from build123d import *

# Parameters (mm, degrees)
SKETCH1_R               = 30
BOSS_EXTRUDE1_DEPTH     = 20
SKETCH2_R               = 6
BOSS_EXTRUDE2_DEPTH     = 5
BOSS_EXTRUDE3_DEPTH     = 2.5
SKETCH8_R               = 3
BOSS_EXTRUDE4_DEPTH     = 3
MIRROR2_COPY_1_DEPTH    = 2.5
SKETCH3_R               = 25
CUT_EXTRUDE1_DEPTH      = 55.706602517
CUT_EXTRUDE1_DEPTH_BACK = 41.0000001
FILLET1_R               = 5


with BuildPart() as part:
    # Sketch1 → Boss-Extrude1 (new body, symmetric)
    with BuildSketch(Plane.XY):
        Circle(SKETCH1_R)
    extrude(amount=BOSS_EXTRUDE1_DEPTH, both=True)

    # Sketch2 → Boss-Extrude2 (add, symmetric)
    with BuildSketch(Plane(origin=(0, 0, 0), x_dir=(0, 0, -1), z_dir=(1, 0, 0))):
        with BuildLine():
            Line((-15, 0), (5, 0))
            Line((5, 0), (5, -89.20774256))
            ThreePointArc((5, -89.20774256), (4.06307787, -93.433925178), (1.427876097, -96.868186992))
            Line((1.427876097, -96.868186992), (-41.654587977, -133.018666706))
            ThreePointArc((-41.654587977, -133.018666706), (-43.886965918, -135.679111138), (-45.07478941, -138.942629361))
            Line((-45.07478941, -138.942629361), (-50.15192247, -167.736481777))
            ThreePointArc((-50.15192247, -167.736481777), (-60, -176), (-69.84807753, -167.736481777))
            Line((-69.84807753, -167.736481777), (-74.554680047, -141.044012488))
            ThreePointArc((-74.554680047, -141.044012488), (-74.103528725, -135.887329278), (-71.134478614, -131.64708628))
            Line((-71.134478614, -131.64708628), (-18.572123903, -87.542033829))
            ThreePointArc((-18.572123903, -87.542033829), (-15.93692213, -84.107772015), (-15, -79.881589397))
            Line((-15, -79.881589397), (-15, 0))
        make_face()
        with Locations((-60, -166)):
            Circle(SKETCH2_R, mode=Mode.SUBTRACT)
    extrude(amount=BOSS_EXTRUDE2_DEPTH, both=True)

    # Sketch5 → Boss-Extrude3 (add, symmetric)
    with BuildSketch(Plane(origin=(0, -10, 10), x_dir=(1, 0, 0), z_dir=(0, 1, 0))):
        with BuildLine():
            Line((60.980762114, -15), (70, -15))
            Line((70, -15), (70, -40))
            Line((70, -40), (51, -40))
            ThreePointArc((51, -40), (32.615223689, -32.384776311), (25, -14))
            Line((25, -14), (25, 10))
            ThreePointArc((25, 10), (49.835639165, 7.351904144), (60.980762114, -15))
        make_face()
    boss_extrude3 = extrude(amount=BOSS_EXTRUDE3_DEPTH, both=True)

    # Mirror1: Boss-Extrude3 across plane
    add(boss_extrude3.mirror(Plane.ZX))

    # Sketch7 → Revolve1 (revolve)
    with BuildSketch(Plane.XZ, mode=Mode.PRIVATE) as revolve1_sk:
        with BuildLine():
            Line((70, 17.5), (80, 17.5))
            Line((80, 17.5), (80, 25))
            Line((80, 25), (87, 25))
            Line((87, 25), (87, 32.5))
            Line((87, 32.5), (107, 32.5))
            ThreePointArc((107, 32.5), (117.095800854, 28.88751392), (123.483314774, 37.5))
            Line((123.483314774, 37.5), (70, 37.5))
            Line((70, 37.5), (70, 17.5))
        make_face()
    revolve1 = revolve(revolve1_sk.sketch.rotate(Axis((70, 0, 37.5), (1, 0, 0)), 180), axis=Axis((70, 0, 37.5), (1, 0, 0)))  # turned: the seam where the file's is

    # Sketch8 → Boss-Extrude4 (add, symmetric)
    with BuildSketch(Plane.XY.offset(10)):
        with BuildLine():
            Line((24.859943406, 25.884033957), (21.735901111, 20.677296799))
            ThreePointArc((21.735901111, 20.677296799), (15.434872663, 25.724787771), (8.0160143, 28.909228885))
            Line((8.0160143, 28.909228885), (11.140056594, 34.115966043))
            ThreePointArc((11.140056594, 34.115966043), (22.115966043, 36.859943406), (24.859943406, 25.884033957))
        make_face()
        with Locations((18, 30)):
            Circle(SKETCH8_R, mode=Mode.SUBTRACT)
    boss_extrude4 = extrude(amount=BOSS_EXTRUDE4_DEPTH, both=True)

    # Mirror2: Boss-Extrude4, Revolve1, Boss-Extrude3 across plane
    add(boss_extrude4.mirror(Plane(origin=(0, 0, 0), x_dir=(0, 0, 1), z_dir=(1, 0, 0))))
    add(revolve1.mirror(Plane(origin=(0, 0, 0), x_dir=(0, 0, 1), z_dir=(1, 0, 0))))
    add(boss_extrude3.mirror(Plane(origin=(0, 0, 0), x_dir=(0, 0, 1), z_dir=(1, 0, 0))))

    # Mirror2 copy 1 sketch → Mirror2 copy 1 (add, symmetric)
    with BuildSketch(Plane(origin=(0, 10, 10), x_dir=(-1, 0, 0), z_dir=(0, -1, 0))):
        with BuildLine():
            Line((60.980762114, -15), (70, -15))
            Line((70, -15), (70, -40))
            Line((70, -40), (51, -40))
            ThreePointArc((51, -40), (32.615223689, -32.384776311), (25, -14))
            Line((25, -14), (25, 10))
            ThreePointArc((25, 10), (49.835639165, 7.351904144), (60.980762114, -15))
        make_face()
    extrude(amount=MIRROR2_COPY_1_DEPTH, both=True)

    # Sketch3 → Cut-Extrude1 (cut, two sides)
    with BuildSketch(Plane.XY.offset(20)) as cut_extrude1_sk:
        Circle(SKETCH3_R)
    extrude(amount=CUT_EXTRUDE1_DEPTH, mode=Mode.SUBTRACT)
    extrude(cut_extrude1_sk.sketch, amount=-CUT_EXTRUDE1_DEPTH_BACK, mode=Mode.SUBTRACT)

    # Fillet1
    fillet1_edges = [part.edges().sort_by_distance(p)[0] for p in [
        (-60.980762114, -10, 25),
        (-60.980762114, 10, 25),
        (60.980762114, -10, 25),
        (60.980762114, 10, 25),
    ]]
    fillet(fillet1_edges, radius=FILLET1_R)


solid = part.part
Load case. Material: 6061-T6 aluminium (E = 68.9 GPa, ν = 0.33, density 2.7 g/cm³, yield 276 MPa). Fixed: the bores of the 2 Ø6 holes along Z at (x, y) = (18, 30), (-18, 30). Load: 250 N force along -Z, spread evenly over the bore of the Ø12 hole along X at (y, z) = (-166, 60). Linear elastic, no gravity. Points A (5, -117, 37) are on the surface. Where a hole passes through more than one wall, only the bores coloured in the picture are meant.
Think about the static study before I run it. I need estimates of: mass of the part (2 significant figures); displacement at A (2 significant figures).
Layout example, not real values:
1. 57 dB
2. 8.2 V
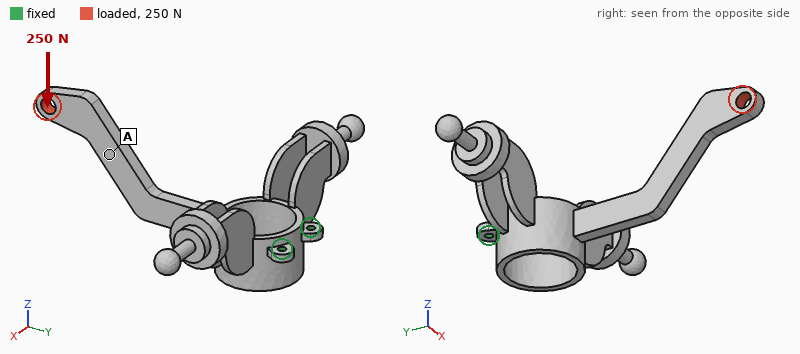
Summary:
1. 400 g
2. 2.1 mm
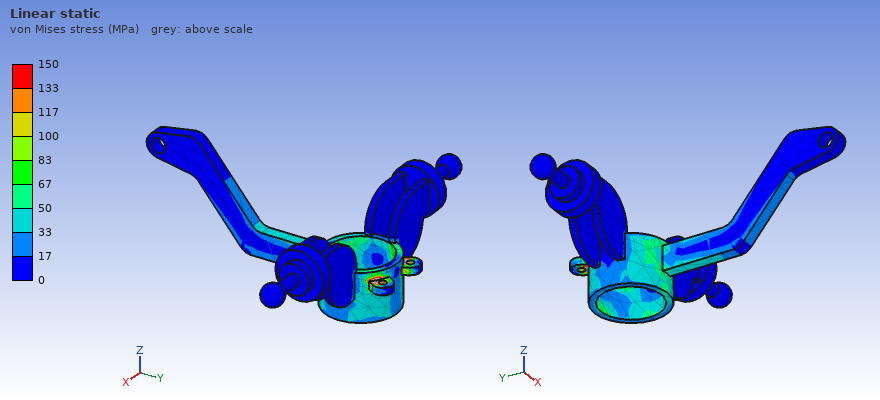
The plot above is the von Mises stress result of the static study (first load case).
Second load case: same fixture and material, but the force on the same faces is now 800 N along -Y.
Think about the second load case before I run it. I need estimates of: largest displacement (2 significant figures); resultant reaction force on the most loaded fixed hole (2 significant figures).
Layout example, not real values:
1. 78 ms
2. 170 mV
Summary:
1. 3.7 mm
2. 400 N
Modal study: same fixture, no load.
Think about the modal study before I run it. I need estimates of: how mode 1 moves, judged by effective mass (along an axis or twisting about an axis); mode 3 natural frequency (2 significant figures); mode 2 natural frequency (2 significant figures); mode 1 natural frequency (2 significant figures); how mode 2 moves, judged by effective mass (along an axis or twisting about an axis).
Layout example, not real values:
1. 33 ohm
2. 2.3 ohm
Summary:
1. along Z
2. 430 Hz
3. 260 Hz
4. 210 Hz
5. along X
